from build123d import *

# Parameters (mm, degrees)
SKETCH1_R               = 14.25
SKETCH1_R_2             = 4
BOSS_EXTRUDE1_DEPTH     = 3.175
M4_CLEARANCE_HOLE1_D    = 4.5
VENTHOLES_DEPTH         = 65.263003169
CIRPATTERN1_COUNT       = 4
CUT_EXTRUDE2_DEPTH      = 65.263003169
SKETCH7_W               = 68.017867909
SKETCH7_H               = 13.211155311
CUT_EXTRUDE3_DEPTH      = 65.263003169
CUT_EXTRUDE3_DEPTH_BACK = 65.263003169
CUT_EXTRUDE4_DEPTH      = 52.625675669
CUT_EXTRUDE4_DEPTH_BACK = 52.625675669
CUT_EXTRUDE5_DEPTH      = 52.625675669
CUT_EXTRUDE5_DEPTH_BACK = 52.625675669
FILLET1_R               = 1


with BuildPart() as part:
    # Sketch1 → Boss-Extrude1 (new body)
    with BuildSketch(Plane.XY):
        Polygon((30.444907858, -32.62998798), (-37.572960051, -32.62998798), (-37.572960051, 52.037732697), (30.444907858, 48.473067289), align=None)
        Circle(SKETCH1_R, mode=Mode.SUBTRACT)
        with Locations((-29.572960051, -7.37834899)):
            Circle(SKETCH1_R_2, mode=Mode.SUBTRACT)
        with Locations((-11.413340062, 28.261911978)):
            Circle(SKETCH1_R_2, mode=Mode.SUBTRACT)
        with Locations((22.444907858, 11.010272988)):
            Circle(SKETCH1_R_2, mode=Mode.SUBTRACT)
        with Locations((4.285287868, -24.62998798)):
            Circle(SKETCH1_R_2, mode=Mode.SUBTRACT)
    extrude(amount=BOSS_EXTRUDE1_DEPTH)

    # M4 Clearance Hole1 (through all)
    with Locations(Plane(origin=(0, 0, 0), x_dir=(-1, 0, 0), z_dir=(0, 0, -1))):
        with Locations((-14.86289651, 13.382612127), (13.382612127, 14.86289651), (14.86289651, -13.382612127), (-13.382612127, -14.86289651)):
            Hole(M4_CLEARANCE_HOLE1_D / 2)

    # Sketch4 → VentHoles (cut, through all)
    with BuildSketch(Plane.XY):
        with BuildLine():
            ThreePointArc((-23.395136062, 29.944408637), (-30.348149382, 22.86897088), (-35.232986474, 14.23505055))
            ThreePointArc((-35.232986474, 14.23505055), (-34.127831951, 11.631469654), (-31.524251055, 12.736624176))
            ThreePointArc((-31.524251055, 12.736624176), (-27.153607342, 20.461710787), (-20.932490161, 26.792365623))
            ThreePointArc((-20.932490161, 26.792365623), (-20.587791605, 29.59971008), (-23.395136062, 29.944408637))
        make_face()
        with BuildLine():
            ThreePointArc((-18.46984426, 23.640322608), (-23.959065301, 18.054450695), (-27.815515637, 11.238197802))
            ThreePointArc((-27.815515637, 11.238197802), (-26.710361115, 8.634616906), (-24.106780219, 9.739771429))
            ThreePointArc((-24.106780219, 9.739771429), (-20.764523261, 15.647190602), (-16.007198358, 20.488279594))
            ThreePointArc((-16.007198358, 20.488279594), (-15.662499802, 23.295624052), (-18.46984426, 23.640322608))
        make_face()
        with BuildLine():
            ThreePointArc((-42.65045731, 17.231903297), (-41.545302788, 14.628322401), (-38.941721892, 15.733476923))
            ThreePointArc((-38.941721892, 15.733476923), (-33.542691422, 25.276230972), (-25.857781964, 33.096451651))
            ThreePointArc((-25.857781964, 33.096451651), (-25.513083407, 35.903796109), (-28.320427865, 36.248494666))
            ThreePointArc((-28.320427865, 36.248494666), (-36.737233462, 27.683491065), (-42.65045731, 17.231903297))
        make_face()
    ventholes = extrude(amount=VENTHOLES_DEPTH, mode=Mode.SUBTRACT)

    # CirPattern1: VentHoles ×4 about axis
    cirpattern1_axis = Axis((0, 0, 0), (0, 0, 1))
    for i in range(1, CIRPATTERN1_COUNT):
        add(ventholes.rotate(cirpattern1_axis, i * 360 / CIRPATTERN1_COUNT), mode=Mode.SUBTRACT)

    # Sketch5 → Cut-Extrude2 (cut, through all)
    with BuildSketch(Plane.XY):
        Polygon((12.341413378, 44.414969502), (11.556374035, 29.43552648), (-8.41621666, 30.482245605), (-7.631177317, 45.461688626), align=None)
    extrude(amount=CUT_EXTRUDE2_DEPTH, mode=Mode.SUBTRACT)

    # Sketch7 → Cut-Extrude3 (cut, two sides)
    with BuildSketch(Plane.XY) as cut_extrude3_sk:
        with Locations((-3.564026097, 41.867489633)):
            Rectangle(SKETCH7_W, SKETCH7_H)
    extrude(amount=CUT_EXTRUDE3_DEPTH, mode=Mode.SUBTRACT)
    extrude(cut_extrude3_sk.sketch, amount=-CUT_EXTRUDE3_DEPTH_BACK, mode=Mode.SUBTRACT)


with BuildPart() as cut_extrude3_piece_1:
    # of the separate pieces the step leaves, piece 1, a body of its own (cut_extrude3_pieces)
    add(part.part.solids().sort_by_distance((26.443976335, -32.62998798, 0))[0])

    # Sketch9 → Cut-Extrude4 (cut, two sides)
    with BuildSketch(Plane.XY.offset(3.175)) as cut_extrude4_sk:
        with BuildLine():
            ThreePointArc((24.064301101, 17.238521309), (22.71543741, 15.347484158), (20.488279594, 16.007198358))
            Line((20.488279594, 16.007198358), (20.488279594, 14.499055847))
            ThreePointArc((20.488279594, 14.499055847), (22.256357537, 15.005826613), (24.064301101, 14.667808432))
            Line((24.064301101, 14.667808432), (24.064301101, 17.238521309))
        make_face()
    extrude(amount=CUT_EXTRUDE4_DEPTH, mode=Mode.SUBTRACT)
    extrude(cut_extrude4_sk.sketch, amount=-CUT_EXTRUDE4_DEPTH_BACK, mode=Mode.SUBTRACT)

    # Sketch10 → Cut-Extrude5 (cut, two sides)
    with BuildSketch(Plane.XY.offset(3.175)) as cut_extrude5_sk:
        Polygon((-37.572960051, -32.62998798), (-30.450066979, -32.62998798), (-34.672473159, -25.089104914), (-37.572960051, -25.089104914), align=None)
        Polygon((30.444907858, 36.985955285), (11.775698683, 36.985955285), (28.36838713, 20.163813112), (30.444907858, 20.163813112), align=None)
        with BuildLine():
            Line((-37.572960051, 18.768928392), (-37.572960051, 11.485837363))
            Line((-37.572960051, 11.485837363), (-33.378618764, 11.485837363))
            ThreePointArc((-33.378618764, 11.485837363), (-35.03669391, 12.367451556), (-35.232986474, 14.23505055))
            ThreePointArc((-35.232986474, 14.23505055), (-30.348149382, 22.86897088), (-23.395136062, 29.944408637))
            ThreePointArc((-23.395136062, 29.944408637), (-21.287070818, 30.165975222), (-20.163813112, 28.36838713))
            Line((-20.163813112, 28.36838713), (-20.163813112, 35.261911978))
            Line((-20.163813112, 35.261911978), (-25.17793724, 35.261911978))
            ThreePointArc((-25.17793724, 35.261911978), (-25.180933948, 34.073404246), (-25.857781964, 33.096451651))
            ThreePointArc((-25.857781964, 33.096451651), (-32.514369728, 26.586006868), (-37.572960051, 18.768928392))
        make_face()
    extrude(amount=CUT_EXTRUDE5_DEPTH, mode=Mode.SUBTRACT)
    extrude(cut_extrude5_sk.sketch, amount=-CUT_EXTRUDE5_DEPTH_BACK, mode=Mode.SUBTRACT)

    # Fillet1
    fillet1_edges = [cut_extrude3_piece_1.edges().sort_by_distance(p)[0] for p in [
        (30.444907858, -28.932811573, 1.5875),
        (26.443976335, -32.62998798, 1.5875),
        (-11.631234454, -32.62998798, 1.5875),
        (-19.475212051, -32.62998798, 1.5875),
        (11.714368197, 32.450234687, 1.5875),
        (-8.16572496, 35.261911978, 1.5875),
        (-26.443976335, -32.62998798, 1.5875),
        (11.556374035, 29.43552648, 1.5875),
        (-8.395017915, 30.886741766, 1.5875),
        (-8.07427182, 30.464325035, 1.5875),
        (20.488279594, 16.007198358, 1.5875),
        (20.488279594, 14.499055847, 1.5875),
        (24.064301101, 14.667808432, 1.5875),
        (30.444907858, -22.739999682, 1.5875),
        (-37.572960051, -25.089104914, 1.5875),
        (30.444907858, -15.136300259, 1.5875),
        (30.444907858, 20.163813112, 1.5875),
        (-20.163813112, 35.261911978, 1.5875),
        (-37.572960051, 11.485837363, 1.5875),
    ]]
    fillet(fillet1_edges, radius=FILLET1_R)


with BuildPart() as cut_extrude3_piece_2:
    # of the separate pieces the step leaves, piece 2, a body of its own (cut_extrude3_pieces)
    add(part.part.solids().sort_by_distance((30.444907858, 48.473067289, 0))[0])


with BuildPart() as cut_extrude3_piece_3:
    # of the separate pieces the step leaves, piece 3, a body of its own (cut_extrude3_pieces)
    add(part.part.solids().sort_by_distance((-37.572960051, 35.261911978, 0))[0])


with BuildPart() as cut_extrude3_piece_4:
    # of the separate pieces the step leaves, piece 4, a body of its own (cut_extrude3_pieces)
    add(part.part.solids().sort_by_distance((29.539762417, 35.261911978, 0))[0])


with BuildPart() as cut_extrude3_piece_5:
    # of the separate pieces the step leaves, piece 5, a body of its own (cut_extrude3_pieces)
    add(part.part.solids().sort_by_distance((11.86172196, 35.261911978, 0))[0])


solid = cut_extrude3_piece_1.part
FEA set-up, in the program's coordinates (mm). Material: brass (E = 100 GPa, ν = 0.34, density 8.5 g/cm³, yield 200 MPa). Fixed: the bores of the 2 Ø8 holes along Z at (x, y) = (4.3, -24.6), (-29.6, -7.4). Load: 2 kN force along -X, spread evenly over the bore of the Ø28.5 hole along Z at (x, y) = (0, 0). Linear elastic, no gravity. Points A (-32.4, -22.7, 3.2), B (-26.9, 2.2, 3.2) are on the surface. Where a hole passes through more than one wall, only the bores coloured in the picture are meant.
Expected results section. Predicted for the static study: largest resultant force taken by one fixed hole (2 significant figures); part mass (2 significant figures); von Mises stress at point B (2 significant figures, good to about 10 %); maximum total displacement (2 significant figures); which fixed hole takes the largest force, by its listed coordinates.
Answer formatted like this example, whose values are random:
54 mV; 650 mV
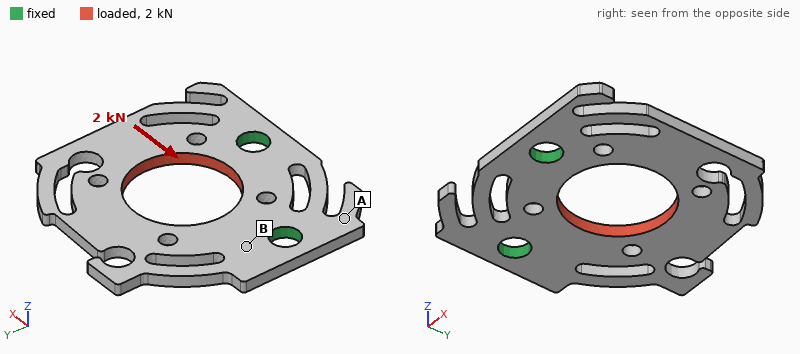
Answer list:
1.2 kN; 72 g; 33 MPa; 37 µm; (-29.6, -7.4)
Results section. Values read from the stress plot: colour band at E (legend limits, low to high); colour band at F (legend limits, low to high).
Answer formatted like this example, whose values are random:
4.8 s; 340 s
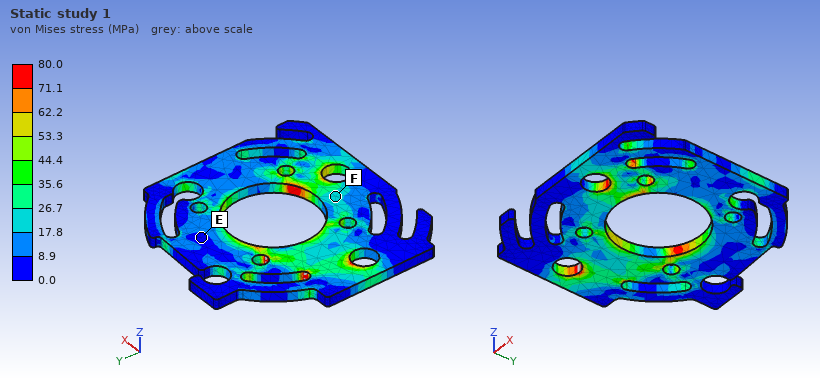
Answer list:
0.0 to 8.9 MPa; 17.8 to 26.7 MPa
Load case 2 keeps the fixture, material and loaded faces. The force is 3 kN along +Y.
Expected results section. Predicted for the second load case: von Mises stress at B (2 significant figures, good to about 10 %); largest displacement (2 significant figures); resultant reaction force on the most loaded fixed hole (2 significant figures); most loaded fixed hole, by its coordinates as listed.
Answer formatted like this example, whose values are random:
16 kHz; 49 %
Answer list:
11 MPa; 41 µm; 2.2 kN; (4.3, -24.6)
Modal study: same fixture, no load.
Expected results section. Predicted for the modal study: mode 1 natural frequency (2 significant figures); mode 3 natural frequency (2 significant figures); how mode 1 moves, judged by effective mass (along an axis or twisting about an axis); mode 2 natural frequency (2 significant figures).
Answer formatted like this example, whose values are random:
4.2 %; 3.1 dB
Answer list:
720 Hz; 3100 Hz; along Z; 1600 Hz
